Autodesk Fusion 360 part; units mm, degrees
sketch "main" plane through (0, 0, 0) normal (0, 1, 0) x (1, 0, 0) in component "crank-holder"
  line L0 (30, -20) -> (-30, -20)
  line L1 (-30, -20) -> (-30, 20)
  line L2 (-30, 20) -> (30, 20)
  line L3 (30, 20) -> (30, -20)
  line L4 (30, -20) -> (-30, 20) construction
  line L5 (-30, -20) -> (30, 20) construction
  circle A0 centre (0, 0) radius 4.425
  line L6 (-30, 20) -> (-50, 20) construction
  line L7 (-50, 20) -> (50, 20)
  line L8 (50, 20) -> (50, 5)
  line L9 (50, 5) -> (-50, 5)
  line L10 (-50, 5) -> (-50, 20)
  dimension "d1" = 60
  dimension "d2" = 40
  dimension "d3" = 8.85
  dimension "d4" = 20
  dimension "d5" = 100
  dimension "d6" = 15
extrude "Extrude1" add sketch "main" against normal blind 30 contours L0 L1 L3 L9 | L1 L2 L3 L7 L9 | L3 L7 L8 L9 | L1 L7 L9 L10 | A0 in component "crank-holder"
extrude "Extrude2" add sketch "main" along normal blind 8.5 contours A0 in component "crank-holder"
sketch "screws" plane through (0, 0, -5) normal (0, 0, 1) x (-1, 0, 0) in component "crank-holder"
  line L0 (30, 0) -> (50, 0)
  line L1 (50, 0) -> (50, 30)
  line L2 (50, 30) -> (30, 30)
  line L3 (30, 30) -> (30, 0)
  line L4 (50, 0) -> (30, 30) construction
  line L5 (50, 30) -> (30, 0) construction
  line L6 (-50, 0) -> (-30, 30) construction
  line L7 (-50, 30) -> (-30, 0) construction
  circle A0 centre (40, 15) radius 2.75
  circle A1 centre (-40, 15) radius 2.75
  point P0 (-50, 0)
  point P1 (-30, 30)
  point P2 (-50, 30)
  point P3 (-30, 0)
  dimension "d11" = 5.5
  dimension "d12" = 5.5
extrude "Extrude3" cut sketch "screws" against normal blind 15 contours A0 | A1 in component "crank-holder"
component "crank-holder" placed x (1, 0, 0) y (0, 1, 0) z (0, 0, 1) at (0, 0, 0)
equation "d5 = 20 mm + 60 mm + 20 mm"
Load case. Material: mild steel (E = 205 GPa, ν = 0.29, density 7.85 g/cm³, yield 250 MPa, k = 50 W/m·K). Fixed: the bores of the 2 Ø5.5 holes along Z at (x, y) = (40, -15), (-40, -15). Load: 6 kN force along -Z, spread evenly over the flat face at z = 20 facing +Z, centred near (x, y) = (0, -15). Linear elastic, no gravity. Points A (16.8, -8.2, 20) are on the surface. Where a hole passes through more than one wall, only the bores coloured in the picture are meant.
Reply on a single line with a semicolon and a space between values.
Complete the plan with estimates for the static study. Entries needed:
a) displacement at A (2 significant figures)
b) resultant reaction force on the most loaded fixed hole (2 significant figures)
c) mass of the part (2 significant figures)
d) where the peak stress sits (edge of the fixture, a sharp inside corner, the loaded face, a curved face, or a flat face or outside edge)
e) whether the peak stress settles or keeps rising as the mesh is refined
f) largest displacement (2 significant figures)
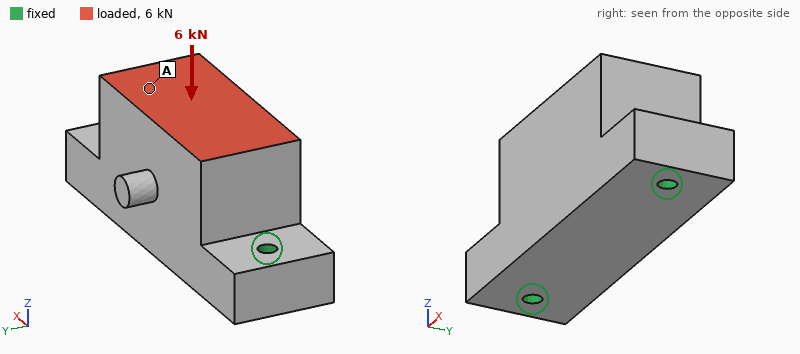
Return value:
3.4 µm; 3.2 kN; 710 g; edge of the fixture; keeps rising; 3.7 µm
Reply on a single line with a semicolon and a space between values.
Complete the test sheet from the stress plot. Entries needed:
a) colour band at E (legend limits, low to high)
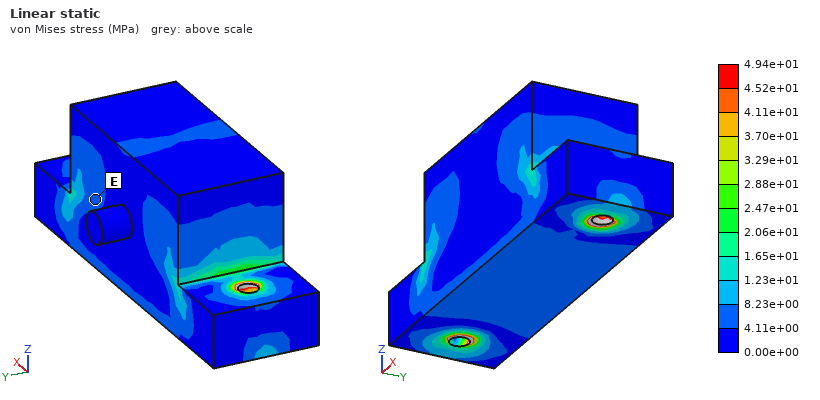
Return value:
4.11e+00 to 8.23e+00 MPa
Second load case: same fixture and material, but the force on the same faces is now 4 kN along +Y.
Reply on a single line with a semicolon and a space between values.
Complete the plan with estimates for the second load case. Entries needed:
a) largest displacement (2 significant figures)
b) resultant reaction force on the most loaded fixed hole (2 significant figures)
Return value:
26 µm; 2.0 kN
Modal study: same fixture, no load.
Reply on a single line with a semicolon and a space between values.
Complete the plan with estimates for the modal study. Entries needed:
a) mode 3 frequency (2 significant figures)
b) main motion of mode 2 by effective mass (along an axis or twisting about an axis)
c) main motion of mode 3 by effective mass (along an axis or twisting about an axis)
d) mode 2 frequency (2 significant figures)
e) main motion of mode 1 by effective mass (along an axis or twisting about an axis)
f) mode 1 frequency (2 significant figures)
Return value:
11 kHz; along Z; along Y; 9000 Hz; along Y; 4600 Hz
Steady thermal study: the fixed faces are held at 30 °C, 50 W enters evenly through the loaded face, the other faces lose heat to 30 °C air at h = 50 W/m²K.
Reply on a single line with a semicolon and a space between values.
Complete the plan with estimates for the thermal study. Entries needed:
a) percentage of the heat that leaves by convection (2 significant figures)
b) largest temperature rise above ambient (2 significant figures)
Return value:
20 %; 33 K
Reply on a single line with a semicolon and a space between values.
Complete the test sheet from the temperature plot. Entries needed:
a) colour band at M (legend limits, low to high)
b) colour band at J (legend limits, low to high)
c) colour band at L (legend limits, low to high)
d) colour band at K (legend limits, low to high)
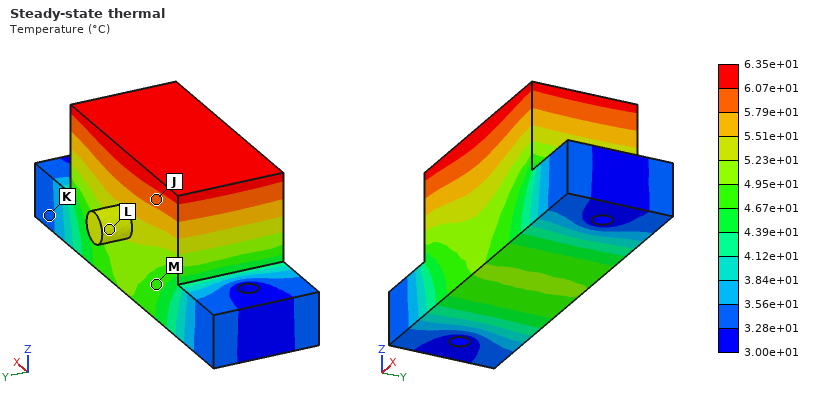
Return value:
4.67e+01 to 4.95e+01 °C; 5.79e+01 to 6.07e+01 °C; 5.23e+01 to 5.51e+01 °C; 3.28e+01 to 3.56e+01 °C
